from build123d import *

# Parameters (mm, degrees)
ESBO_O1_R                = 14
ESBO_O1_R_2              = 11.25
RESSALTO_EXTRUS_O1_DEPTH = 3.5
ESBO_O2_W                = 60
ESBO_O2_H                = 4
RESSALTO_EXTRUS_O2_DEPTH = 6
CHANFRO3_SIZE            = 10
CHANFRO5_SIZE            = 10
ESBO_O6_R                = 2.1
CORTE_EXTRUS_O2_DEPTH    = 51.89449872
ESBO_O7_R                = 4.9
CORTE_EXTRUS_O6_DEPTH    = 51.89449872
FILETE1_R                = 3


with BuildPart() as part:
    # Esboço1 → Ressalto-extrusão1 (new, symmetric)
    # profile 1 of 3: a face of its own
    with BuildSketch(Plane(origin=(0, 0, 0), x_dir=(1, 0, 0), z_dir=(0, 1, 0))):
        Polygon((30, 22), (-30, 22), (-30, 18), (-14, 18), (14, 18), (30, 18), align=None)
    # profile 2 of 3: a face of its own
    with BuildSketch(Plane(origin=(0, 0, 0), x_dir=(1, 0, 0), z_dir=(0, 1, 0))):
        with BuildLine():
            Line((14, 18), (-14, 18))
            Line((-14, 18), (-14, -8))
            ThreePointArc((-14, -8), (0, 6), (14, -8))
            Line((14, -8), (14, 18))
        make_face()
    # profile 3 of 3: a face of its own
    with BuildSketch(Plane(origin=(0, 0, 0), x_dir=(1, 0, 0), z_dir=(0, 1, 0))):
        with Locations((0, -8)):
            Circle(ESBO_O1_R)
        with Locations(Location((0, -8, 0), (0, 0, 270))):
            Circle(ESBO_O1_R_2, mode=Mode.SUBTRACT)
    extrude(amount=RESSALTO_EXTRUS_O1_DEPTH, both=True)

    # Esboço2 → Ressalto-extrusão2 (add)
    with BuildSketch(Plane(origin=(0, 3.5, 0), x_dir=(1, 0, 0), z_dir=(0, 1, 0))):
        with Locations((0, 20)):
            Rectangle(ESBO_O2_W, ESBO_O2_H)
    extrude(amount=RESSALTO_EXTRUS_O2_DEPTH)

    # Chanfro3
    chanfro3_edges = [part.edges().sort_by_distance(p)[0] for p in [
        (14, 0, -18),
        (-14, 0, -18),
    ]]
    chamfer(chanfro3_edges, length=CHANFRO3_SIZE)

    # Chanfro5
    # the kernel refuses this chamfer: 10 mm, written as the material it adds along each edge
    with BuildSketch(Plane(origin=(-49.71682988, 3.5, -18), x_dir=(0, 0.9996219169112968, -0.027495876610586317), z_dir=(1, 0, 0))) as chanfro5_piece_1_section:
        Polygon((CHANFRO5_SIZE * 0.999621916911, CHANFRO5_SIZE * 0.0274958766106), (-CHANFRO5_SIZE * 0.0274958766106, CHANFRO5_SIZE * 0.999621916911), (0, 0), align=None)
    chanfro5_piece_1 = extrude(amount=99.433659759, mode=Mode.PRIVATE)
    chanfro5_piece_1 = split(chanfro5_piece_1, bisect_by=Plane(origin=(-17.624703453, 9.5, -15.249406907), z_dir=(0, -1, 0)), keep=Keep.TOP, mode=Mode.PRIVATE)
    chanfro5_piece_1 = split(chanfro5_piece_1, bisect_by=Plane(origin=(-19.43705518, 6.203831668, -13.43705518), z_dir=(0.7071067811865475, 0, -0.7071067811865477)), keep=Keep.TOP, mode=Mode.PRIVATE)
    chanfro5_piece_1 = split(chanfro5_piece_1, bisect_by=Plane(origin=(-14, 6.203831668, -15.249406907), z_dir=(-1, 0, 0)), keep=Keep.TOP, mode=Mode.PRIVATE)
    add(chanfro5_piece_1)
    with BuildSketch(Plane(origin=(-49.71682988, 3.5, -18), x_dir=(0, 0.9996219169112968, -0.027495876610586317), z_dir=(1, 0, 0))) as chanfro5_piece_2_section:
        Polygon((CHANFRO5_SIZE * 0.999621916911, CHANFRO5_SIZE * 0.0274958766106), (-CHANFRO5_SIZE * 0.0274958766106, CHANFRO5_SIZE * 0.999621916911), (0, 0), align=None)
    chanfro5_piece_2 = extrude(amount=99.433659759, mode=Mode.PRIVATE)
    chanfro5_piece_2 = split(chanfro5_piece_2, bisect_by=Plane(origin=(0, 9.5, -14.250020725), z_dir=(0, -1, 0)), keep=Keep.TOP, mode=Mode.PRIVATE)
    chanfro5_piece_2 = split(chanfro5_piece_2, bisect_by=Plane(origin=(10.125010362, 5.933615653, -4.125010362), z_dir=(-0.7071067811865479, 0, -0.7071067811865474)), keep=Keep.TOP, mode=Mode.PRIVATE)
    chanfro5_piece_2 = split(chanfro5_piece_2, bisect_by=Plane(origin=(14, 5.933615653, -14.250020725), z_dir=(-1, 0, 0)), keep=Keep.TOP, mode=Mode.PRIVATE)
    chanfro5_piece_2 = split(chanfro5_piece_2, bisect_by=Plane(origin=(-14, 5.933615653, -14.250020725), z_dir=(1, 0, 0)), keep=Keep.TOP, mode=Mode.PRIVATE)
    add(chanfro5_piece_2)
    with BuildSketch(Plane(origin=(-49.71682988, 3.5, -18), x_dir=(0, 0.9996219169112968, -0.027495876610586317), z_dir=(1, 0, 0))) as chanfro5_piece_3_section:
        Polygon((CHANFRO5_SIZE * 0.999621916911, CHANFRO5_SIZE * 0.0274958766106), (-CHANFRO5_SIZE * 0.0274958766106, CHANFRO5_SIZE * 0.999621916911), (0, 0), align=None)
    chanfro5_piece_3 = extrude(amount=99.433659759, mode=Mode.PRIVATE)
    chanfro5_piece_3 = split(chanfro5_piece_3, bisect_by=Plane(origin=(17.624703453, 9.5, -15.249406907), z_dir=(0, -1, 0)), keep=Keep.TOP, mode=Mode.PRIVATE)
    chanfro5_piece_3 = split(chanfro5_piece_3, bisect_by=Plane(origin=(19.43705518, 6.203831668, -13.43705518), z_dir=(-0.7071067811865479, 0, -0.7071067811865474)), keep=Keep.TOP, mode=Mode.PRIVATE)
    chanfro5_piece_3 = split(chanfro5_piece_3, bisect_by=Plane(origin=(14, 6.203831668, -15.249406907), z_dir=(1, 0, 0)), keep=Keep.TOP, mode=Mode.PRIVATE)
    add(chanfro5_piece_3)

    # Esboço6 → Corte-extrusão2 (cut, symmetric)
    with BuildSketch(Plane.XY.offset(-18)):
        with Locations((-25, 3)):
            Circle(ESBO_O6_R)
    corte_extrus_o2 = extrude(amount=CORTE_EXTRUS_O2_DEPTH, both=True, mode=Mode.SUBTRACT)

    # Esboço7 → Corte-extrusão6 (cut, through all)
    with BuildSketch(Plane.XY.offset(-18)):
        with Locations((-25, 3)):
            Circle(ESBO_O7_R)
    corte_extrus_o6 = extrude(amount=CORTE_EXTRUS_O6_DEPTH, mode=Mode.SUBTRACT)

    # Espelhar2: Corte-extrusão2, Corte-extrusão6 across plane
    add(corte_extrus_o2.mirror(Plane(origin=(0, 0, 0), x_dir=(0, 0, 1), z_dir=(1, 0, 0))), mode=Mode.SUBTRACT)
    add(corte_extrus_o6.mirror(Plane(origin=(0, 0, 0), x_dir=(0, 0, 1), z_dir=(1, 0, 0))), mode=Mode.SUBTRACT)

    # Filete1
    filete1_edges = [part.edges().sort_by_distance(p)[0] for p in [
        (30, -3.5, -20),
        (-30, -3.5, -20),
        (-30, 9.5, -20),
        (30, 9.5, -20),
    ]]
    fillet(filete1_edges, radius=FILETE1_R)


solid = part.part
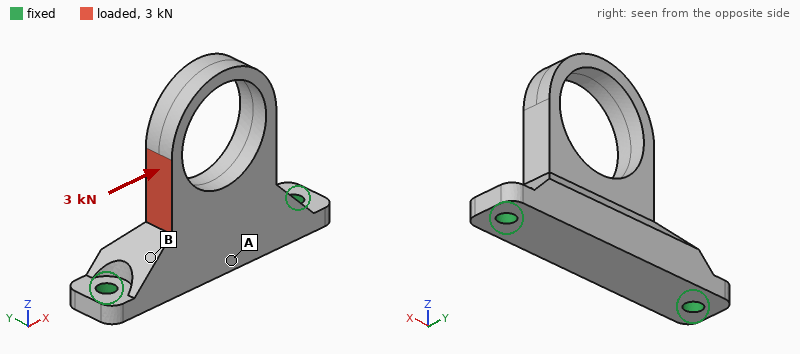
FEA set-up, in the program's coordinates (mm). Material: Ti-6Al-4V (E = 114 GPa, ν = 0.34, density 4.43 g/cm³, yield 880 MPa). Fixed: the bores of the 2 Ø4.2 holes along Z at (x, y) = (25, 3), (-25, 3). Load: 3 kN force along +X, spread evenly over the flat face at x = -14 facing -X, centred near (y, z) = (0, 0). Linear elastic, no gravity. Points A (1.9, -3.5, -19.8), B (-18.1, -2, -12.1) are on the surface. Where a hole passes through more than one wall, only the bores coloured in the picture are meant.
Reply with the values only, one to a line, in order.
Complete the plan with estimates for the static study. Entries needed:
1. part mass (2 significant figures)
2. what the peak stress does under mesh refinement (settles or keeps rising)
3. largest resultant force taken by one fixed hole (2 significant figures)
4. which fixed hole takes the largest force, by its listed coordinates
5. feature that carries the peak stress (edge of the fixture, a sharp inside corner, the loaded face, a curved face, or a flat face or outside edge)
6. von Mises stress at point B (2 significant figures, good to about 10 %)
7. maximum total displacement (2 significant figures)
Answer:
43 g
keeps rising
2.2 kN
(25, 3)
edge of the fixture
48 MPa
66 µm
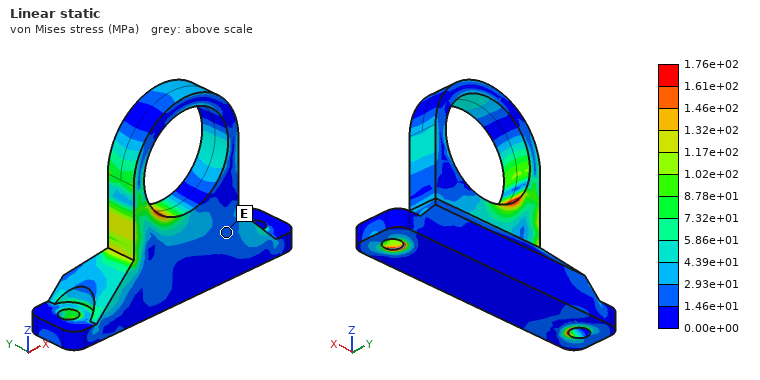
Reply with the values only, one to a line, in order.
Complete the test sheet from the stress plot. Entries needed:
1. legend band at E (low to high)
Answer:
1.46e+01 to 2.93e+01 MPa
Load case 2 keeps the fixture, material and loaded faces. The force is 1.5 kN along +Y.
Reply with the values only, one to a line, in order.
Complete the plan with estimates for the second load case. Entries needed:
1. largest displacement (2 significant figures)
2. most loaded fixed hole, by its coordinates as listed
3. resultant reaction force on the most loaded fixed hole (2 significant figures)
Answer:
0.29 mm
(-25, 3)
1.2 kN
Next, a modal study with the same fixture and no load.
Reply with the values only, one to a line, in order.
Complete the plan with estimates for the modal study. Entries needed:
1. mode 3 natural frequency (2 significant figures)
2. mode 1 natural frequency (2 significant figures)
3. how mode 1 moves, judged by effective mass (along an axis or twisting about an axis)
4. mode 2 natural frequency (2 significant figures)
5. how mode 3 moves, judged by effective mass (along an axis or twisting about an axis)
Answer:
9900 Hz
3600 Hz
along Y
7500 Hz
along Y
